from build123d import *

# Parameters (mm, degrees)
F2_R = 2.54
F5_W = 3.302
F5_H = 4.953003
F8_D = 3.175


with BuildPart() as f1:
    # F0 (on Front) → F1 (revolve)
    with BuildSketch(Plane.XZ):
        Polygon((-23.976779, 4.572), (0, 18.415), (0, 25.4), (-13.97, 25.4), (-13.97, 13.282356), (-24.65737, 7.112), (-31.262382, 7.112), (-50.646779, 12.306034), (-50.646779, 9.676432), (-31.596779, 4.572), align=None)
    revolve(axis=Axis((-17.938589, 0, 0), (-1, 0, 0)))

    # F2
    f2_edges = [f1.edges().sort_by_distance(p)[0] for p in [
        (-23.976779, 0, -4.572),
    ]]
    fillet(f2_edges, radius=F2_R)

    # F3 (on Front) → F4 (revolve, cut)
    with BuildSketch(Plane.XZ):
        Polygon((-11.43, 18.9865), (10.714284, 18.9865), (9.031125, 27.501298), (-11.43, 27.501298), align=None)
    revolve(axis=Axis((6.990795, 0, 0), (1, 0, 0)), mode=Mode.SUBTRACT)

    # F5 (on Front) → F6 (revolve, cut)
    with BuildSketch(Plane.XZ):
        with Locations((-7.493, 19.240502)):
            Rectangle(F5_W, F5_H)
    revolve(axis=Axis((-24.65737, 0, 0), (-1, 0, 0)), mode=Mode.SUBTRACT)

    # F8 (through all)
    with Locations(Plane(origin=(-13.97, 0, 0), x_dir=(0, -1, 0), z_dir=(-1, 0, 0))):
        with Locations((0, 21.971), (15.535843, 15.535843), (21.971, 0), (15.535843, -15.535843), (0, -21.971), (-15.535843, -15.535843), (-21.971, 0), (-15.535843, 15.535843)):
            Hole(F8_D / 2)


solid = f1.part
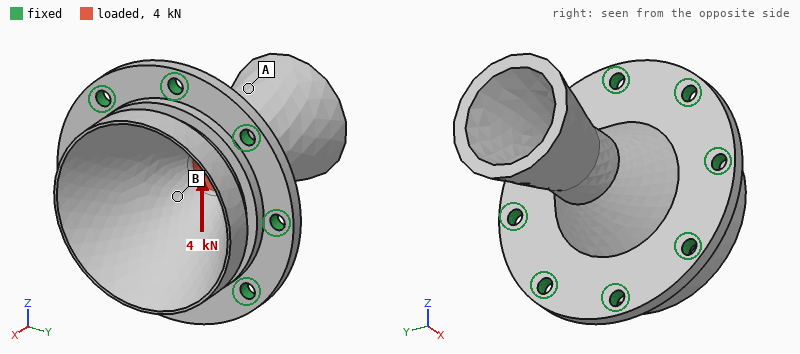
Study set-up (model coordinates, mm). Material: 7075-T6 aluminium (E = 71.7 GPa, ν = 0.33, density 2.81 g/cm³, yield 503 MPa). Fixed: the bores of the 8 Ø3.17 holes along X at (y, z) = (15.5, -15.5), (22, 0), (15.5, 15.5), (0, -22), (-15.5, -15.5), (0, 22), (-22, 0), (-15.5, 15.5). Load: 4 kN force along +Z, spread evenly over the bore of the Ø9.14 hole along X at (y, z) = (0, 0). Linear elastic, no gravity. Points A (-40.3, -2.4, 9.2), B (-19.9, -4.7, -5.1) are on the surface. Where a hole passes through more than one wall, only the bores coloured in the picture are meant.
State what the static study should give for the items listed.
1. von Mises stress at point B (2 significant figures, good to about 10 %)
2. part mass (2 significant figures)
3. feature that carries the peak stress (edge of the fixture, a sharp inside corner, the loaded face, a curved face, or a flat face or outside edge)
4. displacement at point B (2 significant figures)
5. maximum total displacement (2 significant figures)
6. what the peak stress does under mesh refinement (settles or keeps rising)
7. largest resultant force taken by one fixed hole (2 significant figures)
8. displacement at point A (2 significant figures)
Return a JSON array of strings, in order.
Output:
["56 MPa", "36 g", "edge of the fixture", "0.023 mm", "0.11 mm", "keeps rising", "970 N", "0.088 mm"]
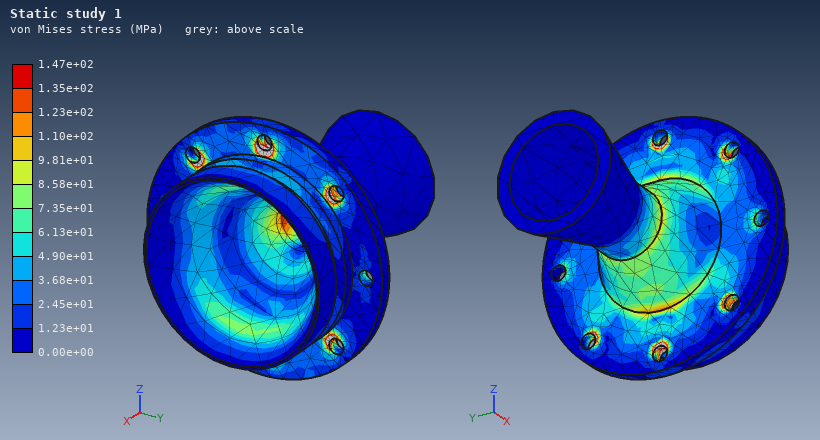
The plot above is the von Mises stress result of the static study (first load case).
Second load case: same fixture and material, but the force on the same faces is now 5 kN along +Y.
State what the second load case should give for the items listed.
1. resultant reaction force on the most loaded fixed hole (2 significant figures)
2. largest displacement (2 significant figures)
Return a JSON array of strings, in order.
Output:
["1.2 kN", "0.14 mm"]
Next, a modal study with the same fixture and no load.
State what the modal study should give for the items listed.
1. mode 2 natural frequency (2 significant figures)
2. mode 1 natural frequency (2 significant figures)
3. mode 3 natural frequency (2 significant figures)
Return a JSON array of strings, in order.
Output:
["6300 Hz", "6300 Hz", "15 kHz"]
